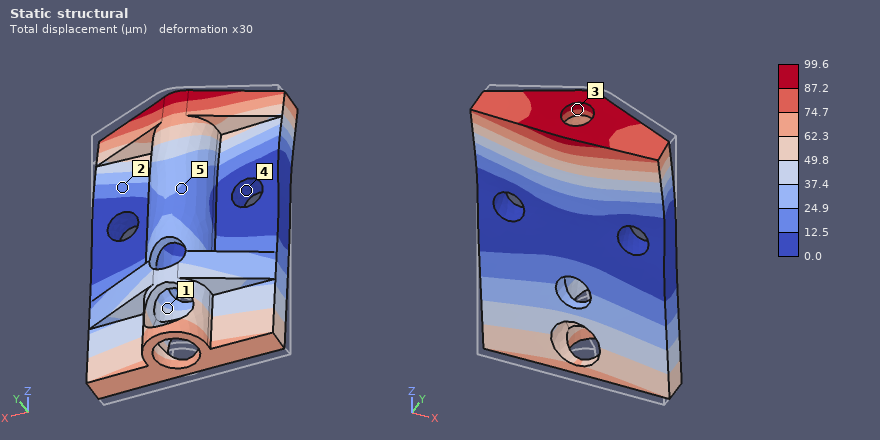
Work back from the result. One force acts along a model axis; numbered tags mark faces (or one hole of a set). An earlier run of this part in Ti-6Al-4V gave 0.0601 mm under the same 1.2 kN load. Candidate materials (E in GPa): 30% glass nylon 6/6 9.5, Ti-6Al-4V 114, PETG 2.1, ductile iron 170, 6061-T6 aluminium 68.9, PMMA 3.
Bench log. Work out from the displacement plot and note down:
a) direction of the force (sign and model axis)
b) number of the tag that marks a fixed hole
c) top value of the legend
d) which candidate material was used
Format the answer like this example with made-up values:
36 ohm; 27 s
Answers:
-Y; 4; 99.6 µm; 6061-T6 aluminium
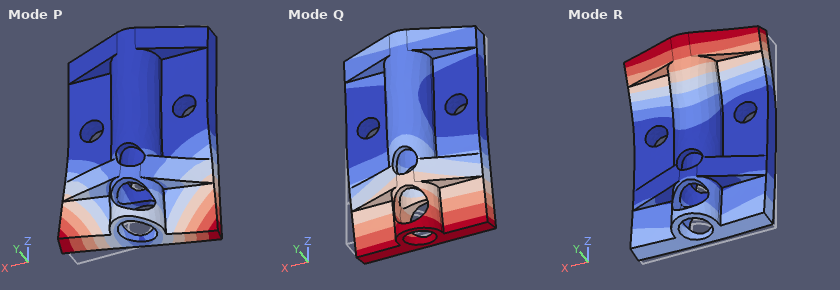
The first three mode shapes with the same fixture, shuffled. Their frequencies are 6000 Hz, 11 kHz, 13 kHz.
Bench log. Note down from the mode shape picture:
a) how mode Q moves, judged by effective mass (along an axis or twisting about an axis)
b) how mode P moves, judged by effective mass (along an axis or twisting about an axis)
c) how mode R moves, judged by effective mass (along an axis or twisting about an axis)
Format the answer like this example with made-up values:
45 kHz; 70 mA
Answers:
along Y; twisting about Z; along Y
